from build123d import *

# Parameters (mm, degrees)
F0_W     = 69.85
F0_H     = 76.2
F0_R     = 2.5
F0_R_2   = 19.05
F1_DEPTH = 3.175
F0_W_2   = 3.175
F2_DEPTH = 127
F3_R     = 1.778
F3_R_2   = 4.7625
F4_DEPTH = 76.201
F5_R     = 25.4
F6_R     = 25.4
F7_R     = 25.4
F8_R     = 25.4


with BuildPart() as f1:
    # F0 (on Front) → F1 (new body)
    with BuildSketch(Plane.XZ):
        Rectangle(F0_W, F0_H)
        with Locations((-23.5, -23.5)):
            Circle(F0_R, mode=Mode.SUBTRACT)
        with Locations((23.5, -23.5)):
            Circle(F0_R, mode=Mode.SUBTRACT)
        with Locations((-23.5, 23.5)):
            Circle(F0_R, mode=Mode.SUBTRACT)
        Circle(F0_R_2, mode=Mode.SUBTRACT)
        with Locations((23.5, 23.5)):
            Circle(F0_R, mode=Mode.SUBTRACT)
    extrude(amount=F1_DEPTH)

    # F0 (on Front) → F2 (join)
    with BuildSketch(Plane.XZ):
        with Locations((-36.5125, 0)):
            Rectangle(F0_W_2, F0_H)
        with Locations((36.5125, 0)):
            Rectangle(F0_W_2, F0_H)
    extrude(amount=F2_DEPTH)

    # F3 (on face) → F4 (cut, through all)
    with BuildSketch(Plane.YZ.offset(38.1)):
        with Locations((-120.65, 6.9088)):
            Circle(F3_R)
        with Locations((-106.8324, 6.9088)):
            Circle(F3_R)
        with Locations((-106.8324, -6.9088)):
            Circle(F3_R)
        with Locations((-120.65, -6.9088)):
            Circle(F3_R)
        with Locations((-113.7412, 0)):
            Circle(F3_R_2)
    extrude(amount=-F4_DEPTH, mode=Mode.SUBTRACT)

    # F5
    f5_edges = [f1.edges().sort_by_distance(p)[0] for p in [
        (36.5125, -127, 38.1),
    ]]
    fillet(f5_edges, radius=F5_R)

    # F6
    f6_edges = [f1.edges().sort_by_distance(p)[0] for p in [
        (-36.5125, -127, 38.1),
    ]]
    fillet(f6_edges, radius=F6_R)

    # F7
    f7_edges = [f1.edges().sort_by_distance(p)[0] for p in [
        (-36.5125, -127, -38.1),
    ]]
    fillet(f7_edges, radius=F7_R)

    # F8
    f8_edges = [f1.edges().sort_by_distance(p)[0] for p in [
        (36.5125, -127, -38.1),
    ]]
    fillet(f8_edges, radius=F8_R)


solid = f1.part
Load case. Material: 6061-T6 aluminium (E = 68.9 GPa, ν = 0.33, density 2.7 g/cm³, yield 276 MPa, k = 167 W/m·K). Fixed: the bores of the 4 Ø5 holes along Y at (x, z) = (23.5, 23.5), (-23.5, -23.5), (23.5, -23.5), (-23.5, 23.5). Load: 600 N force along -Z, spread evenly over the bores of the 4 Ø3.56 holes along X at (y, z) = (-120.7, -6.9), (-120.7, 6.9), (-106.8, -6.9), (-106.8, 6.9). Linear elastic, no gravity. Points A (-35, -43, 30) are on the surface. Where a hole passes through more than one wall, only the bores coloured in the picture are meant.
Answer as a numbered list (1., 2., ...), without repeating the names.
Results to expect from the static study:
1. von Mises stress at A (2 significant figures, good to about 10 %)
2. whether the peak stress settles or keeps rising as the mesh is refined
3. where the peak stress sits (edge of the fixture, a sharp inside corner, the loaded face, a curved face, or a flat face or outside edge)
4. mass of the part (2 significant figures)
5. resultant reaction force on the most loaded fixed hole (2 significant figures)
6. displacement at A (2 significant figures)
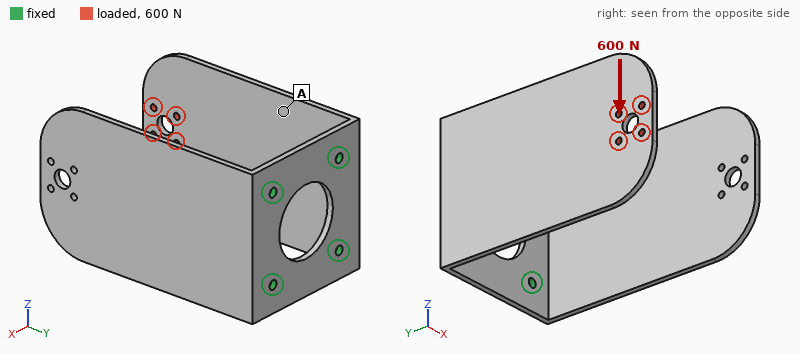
1. 22 MPa
2. keeps rising
3. edge of the fixture
4. 190 g
5. 1.4 kN
6. 0.35 mm
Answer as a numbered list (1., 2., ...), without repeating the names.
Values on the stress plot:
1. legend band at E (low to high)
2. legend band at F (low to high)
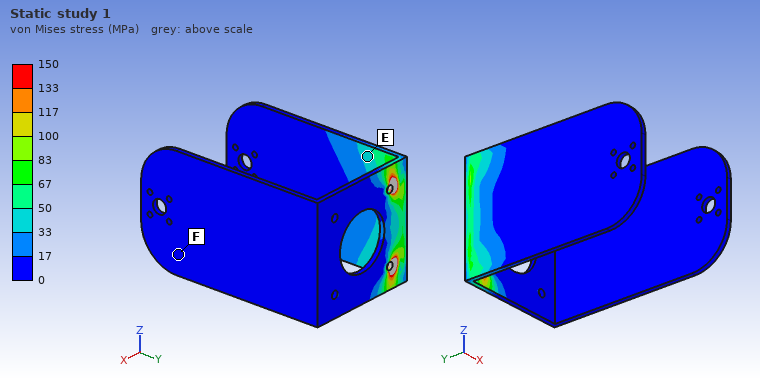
1. 33 to 50 MPa
2. 0 to 17 MPa
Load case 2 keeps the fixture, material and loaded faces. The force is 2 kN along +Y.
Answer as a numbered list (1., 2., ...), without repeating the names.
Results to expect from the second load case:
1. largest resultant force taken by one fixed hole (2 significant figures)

1. 1.0 kN
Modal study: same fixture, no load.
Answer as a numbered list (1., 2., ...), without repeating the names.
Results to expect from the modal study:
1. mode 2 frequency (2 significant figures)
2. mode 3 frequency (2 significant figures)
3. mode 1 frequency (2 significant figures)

1. 150 Hz
2. 600 Hz
3. 150 Hz
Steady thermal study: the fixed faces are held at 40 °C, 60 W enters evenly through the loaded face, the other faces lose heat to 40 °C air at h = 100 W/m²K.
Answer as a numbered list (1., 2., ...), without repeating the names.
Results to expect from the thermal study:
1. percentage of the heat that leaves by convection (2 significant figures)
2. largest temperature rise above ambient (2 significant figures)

1. 88 %
2. 80 K
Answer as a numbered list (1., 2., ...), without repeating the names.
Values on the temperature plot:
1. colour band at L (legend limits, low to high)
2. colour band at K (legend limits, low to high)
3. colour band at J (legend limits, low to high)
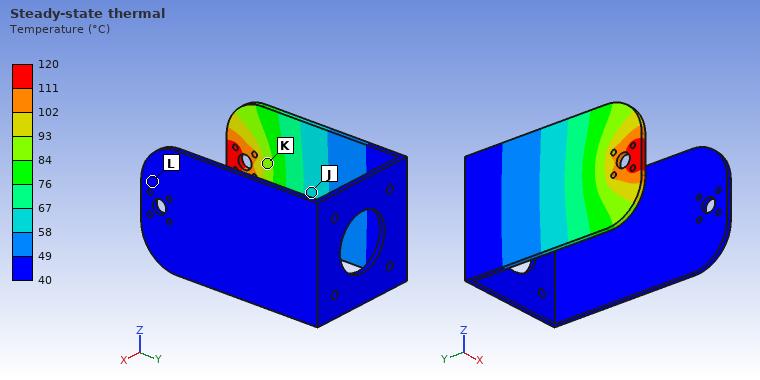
1. 40 to 49 °C
2. 84 to 93 °C
3. 58 to 67 °C
